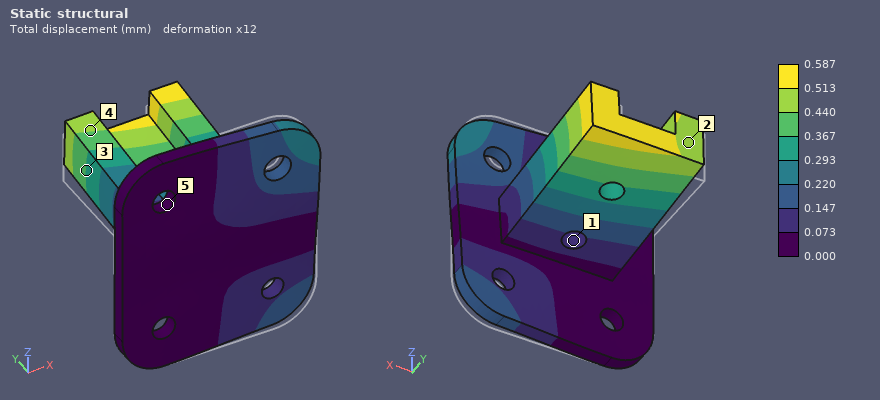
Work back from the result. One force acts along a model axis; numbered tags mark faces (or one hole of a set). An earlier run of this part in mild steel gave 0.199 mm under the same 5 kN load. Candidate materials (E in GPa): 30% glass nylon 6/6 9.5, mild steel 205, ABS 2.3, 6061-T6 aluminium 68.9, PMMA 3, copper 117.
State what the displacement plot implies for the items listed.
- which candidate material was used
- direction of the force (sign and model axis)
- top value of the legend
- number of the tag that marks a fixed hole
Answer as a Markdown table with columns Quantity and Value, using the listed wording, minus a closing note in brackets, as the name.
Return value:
| Quantity | Value |
|---|---|
| which candidate material was used | 6061-T6 aluminium |
| direction of the force | +Z |
| top value of the legend | 0.587 mm |
| number of the tag that marks a fixed hole | 5 |
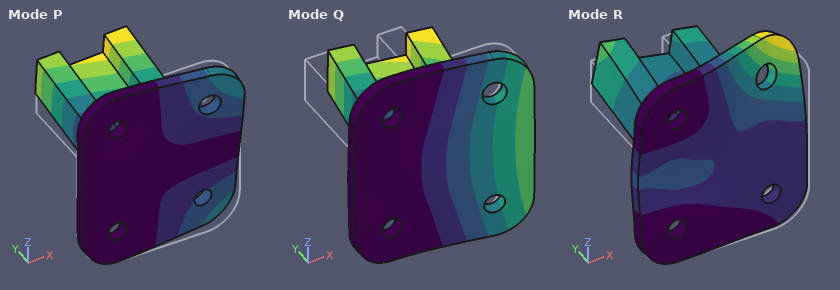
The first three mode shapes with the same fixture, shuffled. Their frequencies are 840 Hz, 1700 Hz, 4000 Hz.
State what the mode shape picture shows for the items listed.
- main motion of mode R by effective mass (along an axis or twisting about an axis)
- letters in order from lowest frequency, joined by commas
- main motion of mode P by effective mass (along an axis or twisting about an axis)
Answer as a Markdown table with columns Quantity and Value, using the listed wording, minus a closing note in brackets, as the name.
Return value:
| Quantity | Value |
|---|---|
| main motion of mode R by effective mass | along Y |
| letters in order from lowest frequency, joined by commas | Q, P, R |
| main motion of mode P by effective mass | along Z |
